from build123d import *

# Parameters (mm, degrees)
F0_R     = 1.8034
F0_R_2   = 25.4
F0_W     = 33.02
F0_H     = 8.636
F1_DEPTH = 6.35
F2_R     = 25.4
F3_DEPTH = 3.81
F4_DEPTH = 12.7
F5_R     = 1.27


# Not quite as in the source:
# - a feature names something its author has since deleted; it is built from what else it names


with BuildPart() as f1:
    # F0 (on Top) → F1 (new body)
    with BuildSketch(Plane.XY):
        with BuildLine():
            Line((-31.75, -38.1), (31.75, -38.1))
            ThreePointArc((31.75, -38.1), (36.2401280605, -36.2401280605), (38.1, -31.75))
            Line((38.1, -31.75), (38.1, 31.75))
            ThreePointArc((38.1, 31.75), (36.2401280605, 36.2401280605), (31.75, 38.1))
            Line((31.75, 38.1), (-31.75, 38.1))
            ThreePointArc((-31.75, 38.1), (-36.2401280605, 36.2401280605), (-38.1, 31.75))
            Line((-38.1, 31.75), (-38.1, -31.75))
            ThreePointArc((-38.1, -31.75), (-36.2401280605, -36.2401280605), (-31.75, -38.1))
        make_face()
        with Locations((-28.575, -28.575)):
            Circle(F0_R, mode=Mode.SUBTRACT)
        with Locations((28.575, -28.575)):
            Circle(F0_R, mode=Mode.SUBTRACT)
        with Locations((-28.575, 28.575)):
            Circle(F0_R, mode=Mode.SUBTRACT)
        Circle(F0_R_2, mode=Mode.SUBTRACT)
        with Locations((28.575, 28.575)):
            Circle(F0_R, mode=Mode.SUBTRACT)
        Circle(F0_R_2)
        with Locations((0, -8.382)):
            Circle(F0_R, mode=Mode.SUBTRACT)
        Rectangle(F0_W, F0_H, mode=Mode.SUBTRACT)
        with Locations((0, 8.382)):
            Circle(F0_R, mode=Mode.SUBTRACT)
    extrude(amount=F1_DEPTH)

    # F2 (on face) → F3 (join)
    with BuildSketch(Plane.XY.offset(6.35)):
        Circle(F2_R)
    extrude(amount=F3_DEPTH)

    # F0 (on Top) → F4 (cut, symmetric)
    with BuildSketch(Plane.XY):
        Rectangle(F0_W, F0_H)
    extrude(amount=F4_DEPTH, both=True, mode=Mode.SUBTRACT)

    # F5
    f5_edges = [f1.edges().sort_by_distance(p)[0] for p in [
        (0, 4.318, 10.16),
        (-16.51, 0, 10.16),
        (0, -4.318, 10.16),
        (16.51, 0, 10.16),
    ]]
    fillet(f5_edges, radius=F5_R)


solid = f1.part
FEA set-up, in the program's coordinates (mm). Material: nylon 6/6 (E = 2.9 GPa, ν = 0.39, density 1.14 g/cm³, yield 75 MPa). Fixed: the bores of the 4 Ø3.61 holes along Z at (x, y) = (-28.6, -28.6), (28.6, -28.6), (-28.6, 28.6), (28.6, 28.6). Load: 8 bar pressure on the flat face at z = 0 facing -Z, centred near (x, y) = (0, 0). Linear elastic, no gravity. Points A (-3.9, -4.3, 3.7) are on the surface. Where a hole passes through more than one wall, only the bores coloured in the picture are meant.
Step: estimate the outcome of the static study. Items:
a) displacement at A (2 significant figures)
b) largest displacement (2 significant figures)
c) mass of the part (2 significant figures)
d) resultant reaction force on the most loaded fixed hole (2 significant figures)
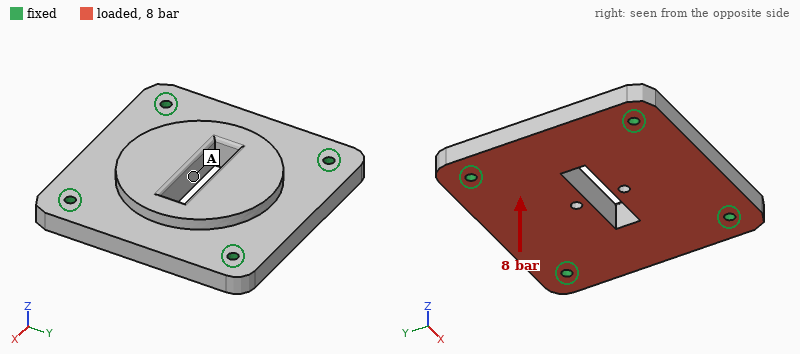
0.72 mm
0.73 mm
47 g
1.1 kN
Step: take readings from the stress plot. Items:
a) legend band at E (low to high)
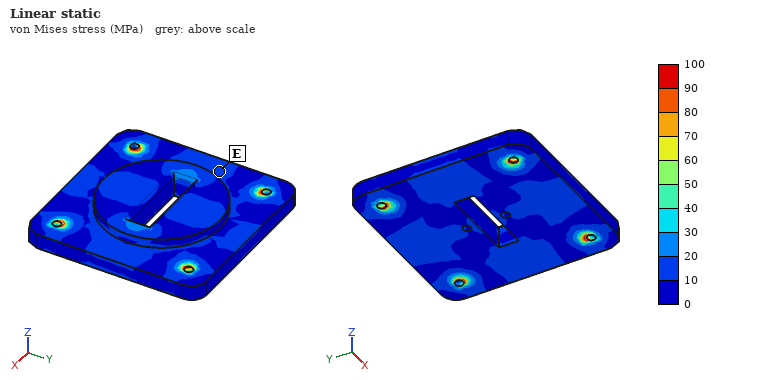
10 to 20 MPa
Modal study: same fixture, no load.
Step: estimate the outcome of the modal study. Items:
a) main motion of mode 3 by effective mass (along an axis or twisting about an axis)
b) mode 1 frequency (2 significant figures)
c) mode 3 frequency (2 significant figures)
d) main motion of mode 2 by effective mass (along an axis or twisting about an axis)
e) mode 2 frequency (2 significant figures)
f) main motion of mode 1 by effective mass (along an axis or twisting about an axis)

twisting about Y
2000 Hz
3200 Hz
twisting about X
3000 Hz
along Z
